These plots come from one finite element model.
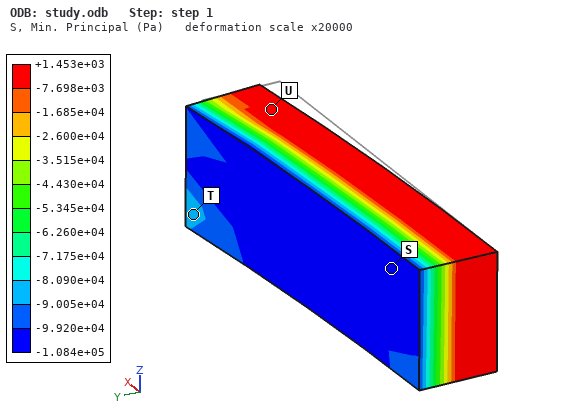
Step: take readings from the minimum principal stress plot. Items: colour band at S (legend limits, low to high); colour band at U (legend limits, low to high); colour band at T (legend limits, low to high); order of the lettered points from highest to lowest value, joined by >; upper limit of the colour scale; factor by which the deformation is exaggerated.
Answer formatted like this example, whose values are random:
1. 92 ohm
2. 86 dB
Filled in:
1. -1.084e+05 to -9.920e+04 Pa
2. -7.698e+03 to +1.453e+03 Pa
3. -9.005e+04 to -8.090e+04 Pa
4. U > T > S
5. +1.453e+03 Pa
6. 20000
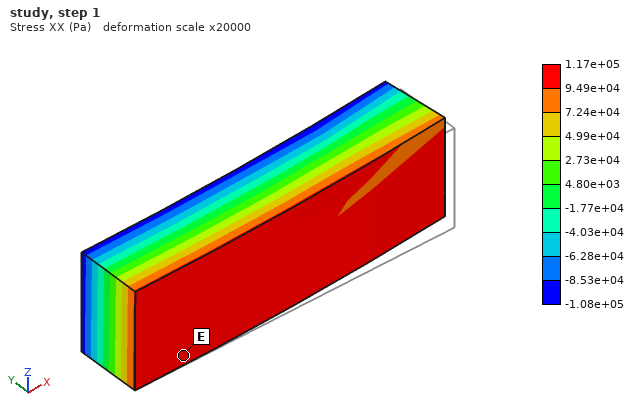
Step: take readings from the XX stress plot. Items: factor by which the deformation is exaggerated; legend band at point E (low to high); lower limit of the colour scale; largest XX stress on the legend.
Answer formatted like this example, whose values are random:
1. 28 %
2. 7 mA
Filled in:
1. 20000
2. 9.49e+04 to 1.17e+05 Pa
3. -1.08e+05 Pa
4. 1.17e+05 Pa
